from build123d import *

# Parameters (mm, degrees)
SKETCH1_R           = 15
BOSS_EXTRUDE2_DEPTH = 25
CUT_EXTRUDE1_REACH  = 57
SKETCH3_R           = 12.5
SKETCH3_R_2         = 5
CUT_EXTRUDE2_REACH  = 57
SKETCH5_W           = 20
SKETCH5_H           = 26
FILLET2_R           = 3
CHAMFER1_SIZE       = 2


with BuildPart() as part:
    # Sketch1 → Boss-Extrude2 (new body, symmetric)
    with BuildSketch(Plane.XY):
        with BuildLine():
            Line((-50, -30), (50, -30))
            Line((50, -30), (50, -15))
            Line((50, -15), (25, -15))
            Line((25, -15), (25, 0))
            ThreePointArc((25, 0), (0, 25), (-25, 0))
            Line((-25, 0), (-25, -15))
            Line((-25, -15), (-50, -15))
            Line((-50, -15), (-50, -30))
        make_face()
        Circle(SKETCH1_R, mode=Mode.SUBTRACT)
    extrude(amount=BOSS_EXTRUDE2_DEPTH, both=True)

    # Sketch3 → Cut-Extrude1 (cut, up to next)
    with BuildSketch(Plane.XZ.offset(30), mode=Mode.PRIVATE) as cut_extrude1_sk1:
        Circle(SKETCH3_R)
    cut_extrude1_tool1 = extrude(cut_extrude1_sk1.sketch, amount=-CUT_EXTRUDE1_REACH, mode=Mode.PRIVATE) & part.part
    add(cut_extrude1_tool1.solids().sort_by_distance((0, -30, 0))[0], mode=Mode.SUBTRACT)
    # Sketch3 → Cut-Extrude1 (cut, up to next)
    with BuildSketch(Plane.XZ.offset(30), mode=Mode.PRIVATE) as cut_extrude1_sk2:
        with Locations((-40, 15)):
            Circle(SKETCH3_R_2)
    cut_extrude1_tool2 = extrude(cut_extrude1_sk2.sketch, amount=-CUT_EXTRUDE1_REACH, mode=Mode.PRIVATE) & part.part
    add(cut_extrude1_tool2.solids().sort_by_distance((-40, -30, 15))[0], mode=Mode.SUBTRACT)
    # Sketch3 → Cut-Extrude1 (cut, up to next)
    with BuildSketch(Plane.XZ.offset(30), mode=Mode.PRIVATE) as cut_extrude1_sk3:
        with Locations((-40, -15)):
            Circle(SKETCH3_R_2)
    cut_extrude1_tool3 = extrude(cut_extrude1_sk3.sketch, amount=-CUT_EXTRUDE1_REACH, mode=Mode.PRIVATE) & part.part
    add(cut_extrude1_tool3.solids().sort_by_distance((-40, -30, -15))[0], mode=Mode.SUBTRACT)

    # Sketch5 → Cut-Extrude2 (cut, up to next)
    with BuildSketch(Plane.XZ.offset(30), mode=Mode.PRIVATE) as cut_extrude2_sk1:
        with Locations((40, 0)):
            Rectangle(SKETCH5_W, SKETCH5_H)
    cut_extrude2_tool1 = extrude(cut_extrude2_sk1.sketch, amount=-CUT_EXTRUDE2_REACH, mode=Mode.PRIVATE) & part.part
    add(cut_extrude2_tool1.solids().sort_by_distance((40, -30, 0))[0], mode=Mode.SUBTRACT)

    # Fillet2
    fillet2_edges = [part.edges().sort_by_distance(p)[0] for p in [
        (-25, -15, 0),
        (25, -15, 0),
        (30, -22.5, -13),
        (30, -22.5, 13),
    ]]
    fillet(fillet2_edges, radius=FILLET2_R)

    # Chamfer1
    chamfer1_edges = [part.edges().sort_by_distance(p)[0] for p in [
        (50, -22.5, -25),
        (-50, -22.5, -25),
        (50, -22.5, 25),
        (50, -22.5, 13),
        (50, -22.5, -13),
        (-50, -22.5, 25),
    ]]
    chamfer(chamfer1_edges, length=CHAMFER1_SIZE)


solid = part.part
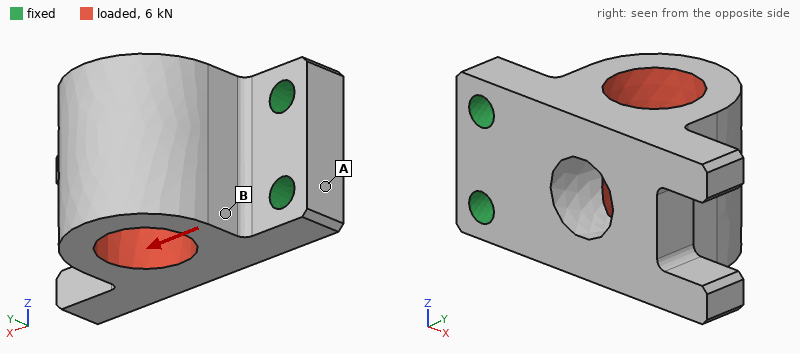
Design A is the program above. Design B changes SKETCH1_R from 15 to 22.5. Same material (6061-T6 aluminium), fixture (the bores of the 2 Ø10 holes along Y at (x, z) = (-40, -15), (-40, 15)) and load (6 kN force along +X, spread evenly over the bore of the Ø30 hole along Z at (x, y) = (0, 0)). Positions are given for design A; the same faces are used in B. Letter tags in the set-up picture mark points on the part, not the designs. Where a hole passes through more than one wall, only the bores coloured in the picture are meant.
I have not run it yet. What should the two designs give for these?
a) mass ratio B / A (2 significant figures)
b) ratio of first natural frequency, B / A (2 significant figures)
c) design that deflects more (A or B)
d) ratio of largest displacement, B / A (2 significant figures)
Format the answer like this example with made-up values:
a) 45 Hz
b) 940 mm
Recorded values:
a) 0.63
b) 0.68
c) B
d) 4.4
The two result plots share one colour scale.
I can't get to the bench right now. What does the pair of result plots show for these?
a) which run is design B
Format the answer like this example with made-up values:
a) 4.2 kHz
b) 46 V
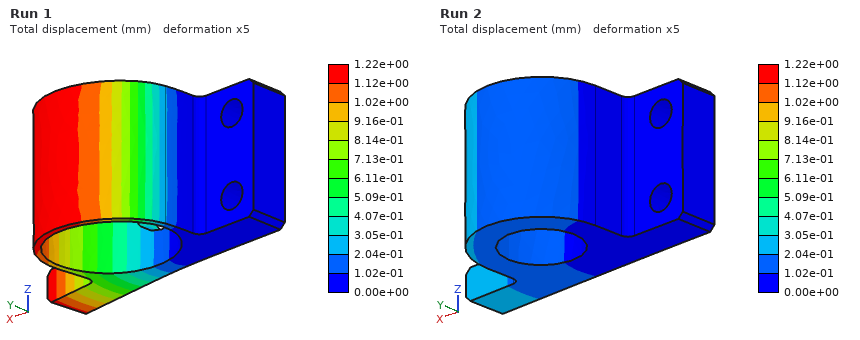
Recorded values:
a) Run 1
